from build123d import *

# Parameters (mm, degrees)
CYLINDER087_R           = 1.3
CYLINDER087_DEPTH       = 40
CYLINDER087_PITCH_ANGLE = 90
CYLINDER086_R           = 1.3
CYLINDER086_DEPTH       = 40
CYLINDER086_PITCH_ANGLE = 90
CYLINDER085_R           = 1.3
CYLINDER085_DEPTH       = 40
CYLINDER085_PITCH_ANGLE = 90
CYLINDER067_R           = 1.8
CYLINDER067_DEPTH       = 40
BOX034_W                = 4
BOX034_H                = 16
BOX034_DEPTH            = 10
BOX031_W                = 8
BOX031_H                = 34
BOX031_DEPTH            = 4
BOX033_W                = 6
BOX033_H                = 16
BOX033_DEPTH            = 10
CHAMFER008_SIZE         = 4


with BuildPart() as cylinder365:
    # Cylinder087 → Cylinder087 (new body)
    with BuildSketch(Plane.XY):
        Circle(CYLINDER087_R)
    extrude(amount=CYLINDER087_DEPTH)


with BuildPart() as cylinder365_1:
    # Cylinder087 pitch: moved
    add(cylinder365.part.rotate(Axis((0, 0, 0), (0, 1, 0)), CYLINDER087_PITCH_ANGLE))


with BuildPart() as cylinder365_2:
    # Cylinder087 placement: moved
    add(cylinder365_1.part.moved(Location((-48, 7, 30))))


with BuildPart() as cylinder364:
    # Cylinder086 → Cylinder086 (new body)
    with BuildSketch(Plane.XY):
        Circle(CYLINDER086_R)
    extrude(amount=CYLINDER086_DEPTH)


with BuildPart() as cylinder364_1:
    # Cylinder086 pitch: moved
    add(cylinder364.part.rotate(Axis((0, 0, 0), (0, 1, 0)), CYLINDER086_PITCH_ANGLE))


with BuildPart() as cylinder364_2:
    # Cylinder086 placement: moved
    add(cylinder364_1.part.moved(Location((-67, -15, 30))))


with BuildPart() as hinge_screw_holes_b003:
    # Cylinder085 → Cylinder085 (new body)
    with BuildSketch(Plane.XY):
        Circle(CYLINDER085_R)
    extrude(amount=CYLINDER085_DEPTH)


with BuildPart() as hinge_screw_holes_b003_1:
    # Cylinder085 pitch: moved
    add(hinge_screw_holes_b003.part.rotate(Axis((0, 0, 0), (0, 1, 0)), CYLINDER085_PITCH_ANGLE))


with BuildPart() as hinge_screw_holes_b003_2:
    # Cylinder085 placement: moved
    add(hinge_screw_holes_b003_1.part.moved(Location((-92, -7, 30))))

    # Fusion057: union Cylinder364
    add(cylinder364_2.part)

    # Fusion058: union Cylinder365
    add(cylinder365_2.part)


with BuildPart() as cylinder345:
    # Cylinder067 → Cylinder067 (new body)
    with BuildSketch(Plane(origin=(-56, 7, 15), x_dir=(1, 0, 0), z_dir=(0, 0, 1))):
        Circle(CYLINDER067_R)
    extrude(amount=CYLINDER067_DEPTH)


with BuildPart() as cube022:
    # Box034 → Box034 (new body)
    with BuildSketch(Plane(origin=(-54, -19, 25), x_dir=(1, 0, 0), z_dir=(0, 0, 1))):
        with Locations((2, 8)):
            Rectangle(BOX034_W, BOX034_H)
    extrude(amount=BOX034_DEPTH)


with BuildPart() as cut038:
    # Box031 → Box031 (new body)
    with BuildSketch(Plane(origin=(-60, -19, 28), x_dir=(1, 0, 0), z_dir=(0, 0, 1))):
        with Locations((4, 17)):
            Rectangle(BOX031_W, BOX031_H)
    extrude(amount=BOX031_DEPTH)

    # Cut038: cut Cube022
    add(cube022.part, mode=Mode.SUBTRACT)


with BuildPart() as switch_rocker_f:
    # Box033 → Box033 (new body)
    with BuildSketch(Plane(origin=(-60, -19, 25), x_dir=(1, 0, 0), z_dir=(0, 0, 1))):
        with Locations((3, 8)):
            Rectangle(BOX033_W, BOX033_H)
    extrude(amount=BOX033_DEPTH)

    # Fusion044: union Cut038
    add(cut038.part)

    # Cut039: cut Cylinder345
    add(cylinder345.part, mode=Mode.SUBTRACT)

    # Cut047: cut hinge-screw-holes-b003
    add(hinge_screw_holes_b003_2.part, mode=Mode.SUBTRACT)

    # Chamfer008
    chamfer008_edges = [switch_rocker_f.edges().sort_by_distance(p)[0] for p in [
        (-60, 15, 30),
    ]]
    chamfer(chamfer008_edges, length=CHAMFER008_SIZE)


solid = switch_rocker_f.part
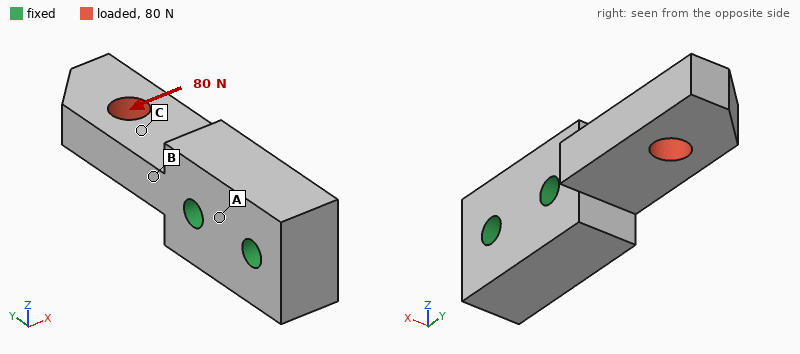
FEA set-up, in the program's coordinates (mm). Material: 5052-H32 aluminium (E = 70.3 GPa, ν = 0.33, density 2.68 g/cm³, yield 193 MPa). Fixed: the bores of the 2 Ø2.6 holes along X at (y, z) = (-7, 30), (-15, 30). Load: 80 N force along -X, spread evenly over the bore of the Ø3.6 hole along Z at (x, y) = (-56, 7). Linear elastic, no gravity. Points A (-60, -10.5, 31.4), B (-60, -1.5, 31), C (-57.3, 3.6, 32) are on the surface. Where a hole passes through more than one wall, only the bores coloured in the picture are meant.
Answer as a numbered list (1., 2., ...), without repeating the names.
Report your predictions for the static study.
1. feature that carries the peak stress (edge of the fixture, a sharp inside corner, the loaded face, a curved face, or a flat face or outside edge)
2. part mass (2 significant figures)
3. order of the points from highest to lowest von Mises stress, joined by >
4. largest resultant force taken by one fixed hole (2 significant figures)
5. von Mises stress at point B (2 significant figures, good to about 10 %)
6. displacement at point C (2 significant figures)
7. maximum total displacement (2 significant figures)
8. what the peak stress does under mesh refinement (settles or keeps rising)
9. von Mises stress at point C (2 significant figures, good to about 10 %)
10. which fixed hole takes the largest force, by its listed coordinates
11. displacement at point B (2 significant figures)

1. edge of the fixture
2. 3.8 g
3. B > C > A
4. 100 N
5. 23 MPa
6. 6.8 µm
7. 19 µm
8. keeps rising
9. 7.3 MPa
10. (-7, 30)
11. 2.9 µm
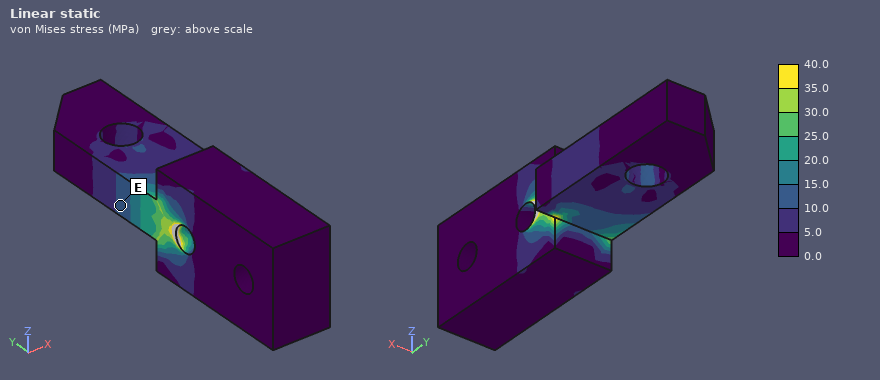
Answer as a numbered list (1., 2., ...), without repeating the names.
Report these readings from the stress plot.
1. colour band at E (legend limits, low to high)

1. 10.0 to 15.0 MPa
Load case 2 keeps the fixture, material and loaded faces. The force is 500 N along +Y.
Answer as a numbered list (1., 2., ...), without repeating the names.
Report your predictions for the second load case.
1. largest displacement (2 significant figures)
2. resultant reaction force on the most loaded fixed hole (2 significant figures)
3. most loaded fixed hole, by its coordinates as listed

1. 9.4 µm
2. 450 N
3. (-7, 30)
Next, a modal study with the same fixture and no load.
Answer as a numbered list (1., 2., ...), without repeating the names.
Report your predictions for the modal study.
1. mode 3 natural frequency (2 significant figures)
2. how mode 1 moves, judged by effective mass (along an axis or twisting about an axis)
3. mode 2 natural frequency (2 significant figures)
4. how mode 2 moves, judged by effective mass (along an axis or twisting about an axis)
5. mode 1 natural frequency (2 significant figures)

1. 31 kHz
2. along Z
3. 12 kHz
4. along X
5. 8600 Hz
